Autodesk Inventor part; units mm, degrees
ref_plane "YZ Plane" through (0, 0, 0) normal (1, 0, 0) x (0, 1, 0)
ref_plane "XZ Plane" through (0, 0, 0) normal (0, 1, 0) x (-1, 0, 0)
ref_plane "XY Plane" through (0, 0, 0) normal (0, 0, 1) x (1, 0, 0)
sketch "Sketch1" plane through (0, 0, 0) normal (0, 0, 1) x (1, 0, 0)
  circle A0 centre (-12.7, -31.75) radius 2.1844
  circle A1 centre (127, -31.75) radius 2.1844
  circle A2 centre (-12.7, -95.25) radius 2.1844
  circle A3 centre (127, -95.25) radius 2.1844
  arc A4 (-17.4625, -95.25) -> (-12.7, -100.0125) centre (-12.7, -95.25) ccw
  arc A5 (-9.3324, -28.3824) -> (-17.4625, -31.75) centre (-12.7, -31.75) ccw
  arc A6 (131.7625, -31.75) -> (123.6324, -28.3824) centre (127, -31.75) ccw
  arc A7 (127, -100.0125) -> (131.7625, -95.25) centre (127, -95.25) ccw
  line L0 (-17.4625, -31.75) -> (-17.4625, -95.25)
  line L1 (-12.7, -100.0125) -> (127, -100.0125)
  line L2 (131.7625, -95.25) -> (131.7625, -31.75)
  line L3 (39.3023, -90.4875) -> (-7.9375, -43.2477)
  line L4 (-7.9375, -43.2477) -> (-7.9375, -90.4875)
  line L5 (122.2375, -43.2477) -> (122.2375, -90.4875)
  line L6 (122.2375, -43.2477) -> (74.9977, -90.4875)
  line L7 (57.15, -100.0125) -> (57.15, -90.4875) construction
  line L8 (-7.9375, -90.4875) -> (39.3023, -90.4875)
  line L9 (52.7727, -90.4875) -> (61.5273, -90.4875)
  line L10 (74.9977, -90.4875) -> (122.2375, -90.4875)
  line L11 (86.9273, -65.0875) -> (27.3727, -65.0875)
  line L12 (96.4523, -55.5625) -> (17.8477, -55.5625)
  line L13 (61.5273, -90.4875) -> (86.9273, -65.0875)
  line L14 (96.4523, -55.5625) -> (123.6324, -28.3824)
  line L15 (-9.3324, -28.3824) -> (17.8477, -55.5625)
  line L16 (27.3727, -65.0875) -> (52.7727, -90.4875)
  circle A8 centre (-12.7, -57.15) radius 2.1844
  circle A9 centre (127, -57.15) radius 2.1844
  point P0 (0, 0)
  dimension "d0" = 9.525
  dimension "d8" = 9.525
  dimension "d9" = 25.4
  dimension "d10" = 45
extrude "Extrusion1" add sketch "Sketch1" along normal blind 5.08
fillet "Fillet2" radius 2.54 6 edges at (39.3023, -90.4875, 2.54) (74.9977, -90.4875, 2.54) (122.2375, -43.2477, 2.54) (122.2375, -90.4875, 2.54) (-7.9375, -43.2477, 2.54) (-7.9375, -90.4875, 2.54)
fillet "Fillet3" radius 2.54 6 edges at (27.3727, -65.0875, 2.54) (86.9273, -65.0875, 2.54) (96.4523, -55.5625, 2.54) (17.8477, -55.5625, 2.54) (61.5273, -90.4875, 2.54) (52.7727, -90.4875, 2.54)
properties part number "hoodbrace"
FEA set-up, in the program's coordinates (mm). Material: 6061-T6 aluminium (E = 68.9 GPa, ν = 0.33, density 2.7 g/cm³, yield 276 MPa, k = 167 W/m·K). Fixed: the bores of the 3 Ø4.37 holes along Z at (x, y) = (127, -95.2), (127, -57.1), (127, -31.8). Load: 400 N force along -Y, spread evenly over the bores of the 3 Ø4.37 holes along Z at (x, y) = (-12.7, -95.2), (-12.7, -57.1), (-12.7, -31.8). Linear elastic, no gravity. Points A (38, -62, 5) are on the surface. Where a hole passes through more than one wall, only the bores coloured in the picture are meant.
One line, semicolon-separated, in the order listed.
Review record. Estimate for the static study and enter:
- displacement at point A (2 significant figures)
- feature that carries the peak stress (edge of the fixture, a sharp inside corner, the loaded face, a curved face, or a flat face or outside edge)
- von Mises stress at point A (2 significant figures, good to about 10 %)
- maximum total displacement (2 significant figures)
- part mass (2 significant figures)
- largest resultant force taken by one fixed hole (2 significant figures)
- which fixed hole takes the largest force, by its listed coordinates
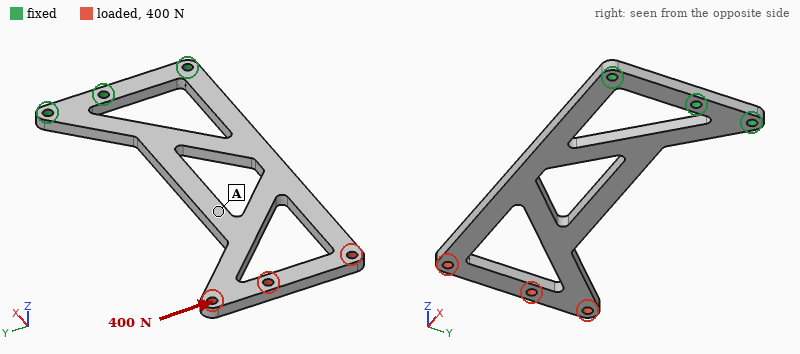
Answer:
0.12 mm; a curved face; 17 MPa; 0.43 mm; 64 g; 1.0 kN; (127, -95.2)
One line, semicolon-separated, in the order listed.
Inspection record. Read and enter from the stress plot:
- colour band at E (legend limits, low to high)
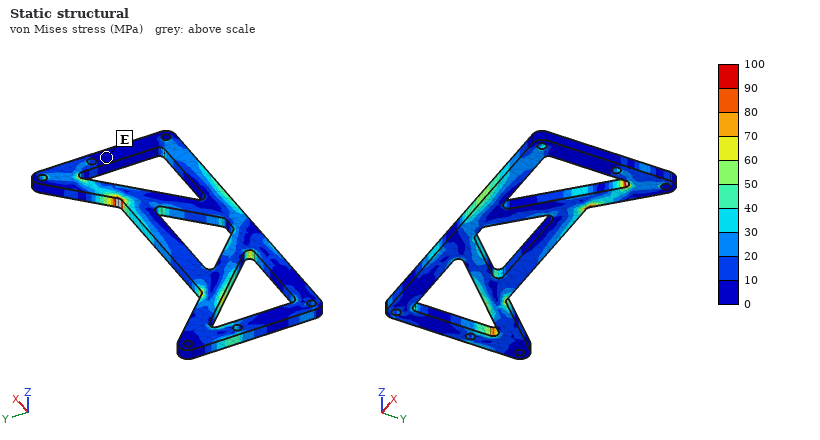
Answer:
0 to 10 MPa
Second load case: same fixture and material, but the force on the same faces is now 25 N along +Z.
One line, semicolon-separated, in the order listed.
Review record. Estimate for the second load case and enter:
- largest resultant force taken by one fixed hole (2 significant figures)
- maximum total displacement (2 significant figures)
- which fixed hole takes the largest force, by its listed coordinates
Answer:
23 N; 1.7 mm; (127, -31.8)
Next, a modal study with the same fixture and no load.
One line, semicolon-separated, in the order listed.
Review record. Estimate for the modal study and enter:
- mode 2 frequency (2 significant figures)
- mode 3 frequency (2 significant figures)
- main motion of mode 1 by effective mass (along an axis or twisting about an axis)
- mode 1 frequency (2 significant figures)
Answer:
650 Hz; 1000 Hz; along Z; 150 Hz
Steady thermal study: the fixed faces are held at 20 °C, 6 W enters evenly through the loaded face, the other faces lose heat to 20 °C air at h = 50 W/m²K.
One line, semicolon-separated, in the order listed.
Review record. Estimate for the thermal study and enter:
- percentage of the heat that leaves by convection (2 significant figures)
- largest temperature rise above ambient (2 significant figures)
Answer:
81 %; 19 K
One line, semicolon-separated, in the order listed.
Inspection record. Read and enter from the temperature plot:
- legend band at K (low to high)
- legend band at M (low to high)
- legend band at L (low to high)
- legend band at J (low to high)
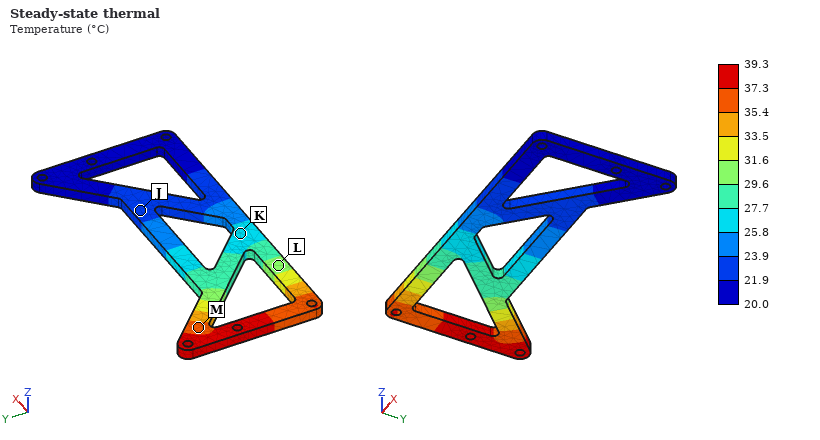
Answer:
25.8 to 27.7 °C; 35.4 to 37.3 °C; 29.6 to 31.6 °C; 21.9 to 23.9 °C
